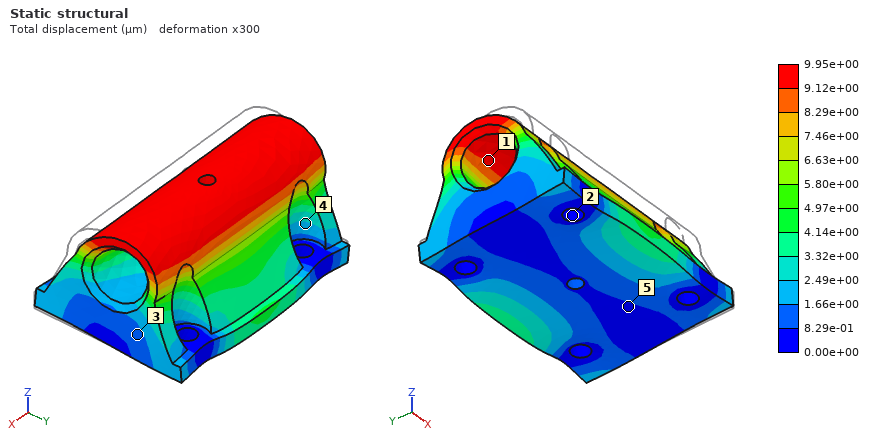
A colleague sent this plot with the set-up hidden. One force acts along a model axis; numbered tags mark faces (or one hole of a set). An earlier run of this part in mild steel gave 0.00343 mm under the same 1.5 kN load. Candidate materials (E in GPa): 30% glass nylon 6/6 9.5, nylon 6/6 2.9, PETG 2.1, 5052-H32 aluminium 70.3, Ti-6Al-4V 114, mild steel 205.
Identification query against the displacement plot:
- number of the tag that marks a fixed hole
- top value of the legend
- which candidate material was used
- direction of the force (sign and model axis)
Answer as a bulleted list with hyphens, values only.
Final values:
- 2
- 9.95e+00 µm
- 5052-H32 aluminium
- +Y
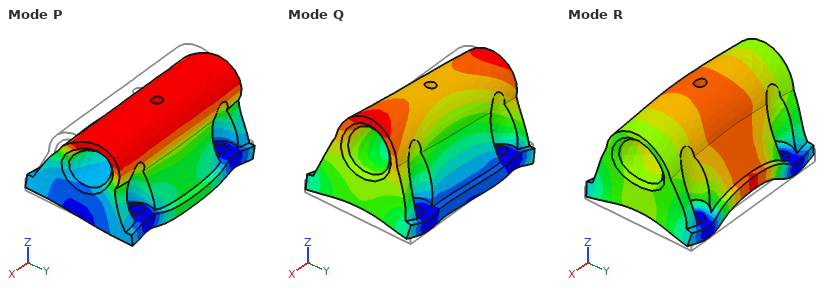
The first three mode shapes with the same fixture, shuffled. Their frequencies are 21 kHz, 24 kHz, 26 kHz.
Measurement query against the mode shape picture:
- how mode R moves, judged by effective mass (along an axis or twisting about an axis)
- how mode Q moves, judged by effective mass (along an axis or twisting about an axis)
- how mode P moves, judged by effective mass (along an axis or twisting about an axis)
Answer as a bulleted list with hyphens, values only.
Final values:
- along Z
- along X
- along Y
